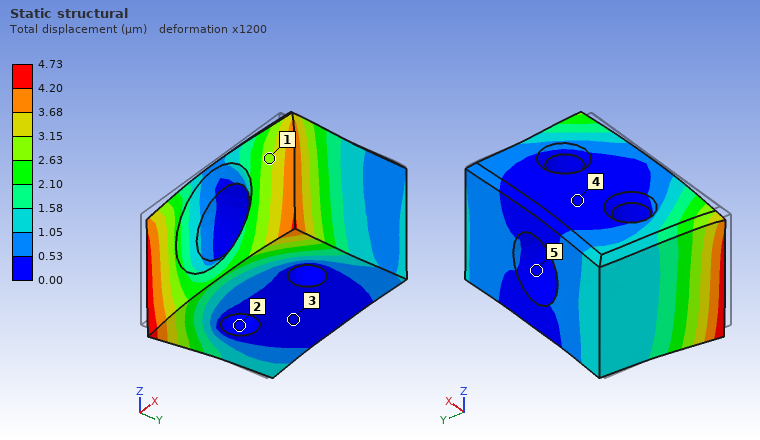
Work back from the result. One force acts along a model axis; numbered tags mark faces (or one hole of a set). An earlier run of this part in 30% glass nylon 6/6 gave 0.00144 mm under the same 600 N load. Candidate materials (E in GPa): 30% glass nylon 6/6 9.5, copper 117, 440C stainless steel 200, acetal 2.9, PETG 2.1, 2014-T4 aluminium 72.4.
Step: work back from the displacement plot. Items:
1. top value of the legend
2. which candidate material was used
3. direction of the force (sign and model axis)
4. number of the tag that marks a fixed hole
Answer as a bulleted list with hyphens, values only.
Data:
- 4.73 µm
- acetal
- +Y
- 2
